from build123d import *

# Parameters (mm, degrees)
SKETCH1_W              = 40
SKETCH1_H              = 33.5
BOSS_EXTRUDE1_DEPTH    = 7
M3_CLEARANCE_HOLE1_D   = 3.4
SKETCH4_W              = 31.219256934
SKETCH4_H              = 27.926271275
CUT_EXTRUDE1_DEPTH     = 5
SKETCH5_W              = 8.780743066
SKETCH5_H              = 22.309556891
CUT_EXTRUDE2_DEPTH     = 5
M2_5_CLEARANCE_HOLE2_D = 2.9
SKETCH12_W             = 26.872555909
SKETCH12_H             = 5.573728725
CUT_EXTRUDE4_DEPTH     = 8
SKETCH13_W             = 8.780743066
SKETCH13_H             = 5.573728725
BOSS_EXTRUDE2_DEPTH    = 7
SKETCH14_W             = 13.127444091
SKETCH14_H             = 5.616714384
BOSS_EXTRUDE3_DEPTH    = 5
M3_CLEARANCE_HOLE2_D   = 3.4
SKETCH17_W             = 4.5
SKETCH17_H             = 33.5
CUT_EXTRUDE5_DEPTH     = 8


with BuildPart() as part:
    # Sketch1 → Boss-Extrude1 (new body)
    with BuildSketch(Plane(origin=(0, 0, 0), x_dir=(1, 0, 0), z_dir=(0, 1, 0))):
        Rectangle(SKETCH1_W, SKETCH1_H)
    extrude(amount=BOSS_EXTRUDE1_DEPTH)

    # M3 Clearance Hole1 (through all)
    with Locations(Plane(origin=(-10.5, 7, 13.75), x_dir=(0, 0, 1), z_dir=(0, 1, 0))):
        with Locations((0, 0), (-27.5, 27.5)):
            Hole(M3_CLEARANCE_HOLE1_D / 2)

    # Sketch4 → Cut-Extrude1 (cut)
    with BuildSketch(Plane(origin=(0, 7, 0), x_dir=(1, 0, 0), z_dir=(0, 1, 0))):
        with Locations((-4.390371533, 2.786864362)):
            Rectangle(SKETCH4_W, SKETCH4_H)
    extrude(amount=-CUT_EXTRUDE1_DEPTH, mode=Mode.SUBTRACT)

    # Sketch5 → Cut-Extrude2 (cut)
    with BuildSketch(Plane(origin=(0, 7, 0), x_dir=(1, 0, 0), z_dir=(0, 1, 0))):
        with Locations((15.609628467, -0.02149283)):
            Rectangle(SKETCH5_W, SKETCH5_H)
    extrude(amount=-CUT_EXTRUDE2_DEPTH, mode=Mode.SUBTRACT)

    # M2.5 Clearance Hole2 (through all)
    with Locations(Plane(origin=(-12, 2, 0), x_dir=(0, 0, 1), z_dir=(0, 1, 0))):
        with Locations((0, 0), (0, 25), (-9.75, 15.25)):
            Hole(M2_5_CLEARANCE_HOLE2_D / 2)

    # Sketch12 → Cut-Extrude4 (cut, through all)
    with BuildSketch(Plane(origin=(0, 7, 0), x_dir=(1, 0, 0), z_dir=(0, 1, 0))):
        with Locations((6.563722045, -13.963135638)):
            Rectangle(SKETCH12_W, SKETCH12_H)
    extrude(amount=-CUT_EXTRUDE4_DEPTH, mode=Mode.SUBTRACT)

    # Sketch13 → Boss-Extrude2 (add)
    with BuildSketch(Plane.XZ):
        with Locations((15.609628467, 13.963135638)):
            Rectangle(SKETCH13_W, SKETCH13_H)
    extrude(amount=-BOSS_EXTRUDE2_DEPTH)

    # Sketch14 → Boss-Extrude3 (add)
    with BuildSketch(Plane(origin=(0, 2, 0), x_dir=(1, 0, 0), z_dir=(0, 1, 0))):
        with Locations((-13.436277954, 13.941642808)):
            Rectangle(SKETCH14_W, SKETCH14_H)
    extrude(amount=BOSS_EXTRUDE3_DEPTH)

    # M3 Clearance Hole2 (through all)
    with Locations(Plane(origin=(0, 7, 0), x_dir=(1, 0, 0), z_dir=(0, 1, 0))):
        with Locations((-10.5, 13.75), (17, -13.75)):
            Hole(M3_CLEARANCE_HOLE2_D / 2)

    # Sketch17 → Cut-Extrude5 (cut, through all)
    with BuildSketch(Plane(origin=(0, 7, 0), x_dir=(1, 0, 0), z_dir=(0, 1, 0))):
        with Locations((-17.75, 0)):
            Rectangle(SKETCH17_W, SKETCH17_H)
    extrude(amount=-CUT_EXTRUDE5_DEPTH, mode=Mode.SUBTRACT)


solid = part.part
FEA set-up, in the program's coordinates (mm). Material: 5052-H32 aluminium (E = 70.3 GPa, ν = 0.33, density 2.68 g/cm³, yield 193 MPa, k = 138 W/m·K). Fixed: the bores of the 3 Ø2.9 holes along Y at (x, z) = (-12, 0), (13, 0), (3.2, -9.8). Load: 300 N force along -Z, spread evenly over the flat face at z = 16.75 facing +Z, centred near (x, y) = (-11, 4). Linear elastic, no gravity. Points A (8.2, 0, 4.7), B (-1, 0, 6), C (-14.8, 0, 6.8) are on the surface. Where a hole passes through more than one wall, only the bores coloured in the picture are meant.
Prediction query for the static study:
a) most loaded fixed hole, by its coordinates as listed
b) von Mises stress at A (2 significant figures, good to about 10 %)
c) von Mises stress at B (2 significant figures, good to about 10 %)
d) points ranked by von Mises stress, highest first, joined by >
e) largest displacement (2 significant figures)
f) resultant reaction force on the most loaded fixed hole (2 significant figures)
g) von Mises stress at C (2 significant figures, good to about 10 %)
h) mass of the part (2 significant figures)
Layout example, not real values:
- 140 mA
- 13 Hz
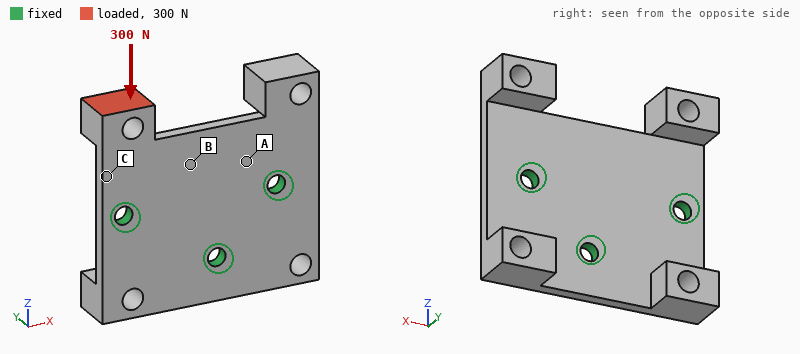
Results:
- (-12, 0)
- 13 MPa
- 34 MPa
- C > B > A
- 0.17 mm
- 270 N
- 75 MPa
- 7.7 g
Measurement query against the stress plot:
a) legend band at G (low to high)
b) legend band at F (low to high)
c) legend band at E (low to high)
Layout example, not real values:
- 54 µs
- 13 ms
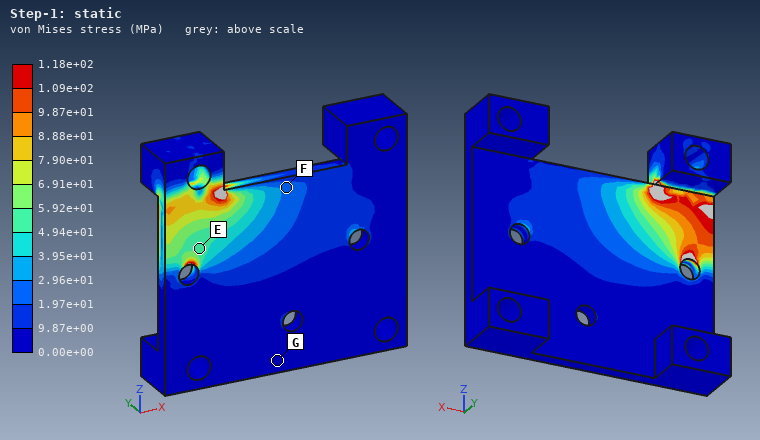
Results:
- 0.00e+00 to 9.87e+00 MPa
- 1.97e+01 to 2.96e+01 MPa
- 4.94e+01 to 5.92e+01 MPa
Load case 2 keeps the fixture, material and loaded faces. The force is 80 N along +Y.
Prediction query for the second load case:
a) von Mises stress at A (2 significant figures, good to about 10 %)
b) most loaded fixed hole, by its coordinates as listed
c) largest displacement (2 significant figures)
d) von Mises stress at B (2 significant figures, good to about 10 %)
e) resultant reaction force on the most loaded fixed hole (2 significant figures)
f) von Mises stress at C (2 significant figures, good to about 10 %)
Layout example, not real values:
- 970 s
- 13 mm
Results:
- 18 MPa
- (-12, 0)
- 0.20 mm
- 45 MPa
- 93 N
- 95 MPa
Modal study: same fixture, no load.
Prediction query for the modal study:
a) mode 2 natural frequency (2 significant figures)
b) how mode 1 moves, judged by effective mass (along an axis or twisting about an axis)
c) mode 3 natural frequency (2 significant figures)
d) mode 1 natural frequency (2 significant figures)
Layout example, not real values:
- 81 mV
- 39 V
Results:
- 4900 Hz
- along Y
- 6700 Hz
- 4500 Hz
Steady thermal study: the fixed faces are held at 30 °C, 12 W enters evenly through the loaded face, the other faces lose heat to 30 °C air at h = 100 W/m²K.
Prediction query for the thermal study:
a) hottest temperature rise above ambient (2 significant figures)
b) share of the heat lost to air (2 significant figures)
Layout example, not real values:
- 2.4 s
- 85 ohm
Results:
- 52 K
- 17 %
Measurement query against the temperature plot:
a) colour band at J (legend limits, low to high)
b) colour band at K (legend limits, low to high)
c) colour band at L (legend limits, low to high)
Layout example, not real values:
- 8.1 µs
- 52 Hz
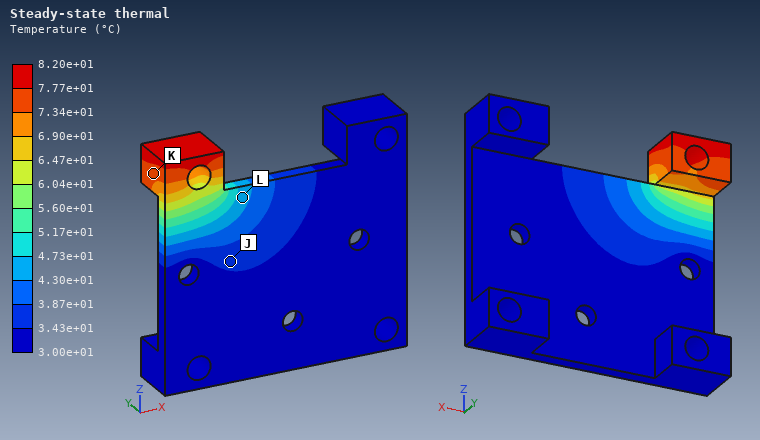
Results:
- 3.43e+01 to 3.87e+01 °C
- 7.34e+01 to 7.77e+01 °C
- 4.30e+01 to 4.73e+01 °C
